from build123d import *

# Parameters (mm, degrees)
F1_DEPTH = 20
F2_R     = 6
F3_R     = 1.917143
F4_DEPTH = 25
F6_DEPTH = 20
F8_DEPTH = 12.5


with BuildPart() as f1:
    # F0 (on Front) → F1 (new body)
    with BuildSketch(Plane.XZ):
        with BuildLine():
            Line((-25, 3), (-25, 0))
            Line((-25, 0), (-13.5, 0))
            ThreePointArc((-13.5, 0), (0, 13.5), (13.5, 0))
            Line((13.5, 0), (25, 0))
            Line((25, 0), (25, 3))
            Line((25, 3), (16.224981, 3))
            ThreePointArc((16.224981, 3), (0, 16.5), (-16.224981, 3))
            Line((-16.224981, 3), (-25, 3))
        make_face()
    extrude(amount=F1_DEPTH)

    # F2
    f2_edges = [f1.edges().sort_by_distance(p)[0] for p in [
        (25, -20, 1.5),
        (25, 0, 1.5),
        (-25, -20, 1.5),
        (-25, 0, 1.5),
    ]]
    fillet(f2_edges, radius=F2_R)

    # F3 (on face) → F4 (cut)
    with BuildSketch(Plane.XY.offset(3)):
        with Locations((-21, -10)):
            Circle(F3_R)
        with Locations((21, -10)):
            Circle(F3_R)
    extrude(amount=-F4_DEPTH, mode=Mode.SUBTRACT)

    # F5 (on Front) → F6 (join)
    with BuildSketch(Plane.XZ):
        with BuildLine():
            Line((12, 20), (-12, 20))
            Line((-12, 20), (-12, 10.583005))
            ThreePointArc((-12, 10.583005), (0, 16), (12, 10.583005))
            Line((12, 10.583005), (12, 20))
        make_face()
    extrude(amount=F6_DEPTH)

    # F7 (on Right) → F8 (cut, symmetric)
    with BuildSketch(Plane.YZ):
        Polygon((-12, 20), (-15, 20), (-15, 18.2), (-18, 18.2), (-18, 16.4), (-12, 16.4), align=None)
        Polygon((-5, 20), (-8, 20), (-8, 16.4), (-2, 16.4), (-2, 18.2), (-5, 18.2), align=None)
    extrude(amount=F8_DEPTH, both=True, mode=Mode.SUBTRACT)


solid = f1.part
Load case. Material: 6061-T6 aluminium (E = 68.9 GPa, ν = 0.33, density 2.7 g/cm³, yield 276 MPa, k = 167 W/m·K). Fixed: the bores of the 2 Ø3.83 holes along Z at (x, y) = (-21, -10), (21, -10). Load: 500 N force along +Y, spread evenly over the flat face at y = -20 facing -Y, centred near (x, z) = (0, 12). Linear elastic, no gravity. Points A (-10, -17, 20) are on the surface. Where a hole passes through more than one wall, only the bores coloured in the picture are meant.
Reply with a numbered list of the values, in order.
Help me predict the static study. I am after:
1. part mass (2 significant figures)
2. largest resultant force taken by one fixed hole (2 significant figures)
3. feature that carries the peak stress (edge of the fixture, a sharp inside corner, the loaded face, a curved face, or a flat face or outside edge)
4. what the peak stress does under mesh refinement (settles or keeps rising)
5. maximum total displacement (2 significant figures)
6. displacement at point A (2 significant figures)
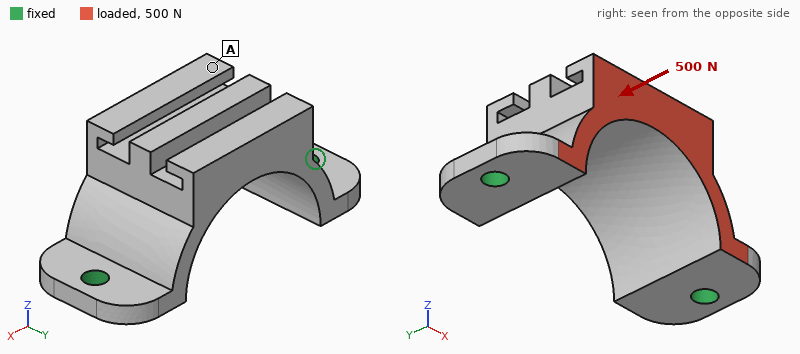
1. 14 g
2. 250 N
3. edge of the fixture
4. keeps rising
5. 80 µm
6. 75 µm
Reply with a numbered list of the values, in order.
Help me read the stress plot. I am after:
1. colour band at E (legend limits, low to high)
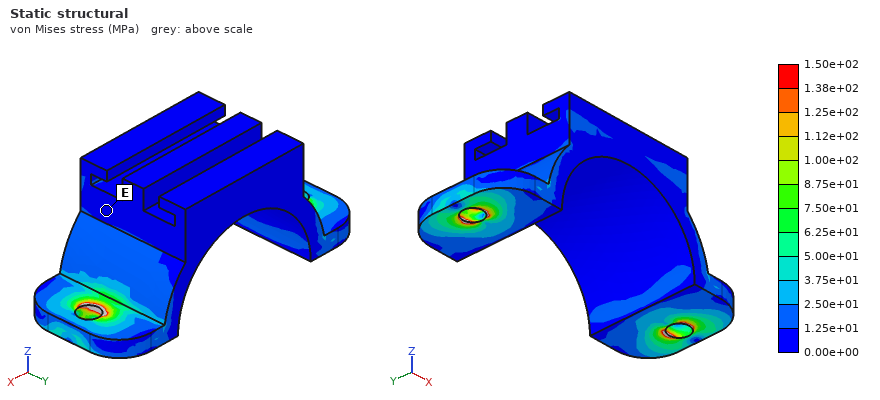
1. 0.00e+00 to 1.25e+01 MPa
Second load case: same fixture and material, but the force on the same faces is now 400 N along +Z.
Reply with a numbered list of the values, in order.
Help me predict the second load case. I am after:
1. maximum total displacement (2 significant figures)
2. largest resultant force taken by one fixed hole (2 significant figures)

1. 54 µm
2. 230 N
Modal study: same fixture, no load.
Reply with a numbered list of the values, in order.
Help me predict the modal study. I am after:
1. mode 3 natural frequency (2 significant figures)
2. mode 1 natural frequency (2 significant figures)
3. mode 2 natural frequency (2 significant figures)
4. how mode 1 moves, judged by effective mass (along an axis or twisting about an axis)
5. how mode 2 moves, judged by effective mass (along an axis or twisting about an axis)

1. 13 kHz
2. 4200 Hz
3. 12 kHz
4. along Y
5. along X
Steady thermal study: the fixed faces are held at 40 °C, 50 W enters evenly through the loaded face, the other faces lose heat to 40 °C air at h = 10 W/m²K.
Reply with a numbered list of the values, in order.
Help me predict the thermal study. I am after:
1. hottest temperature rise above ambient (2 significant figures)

1. 58 K
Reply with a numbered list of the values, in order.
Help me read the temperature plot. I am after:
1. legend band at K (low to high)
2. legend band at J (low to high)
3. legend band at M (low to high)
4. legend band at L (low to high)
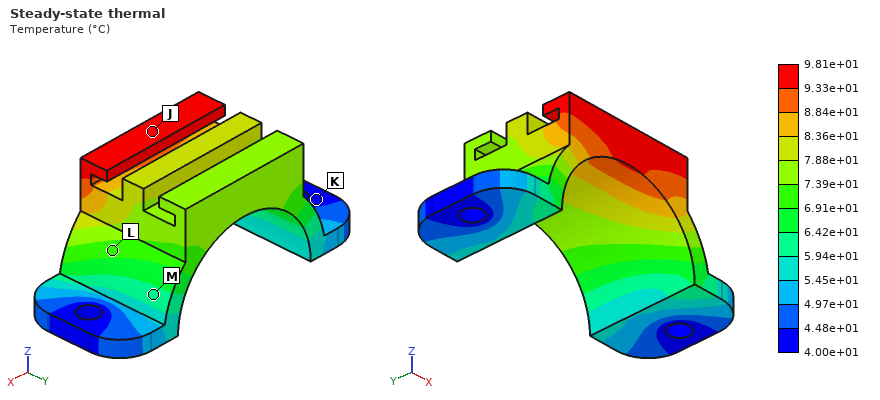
1. 4.00e+01 to 4.48e+01 °C
2. 9.33e+01 to 9.81e+01 °C
3. 5.94e+01 to 6.42e+01 °C
4. 6.91e+01 to 7.39e+01 °C
